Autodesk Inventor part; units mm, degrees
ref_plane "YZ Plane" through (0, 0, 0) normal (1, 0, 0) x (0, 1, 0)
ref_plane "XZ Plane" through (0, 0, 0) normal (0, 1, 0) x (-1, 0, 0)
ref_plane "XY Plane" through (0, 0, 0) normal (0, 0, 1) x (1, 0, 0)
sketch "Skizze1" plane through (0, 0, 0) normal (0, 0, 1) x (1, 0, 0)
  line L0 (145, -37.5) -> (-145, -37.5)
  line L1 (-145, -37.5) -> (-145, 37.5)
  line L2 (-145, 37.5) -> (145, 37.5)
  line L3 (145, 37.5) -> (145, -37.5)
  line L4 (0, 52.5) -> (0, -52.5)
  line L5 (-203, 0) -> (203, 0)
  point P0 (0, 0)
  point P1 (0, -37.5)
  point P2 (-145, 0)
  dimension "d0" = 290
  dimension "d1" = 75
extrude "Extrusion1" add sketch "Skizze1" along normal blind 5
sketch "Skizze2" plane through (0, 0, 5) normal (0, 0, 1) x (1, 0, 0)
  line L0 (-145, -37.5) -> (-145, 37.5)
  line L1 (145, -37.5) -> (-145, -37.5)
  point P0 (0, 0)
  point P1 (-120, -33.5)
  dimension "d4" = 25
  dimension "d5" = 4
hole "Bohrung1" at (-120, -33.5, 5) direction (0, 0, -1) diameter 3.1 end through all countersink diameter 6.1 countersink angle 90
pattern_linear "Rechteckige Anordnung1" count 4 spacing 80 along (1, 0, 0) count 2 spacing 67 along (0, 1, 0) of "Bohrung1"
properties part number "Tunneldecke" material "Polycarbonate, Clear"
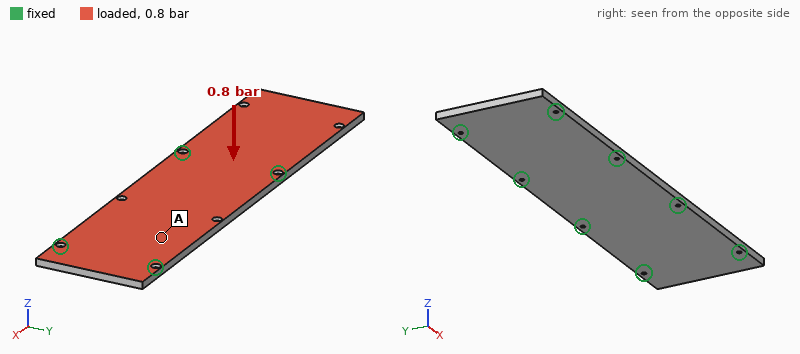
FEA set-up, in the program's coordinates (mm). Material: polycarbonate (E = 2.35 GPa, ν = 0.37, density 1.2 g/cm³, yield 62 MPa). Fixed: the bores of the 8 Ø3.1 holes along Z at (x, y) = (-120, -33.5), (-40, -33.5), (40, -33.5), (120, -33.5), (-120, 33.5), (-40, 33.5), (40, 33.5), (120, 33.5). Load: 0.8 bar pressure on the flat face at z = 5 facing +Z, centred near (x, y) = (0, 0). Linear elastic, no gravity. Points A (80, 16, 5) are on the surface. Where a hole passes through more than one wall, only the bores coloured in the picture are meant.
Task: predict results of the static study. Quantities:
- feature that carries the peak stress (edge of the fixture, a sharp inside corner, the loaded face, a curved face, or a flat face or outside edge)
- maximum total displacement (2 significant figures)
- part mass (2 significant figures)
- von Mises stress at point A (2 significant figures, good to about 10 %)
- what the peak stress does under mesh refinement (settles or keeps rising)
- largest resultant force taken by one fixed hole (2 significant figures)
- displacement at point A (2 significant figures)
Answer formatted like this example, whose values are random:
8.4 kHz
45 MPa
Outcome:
edge of the fixture
0.76 mm
130 g
5.6 MPa
keeps rising
260 N
0.69 mm
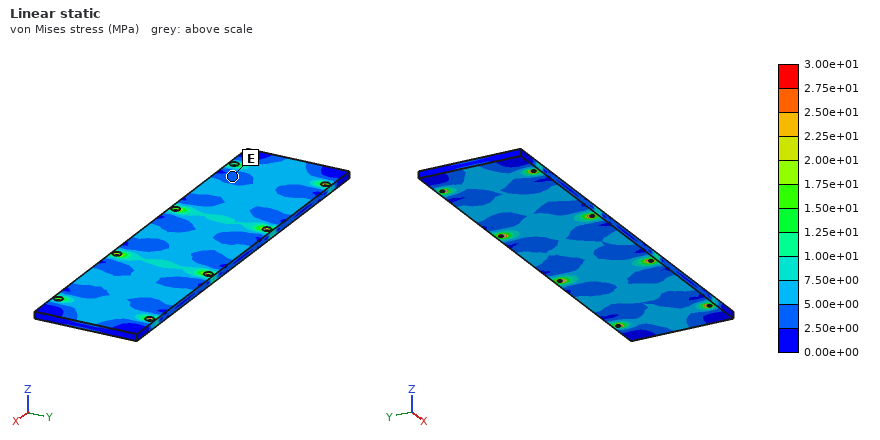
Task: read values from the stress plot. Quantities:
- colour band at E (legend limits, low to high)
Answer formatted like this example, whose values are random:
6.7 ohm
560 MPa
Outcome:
2.50e+00 to 5.00e+00 MPa
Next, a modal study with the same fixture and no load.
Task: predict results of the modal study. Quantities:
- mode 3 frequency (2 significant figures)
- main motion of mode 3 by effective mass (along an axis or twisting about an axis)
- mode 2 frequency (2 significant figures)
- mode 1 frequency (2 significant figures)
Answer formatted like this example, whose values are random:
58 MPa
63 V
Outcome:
780 Hz
along Z
740 Hz
710 Hz
